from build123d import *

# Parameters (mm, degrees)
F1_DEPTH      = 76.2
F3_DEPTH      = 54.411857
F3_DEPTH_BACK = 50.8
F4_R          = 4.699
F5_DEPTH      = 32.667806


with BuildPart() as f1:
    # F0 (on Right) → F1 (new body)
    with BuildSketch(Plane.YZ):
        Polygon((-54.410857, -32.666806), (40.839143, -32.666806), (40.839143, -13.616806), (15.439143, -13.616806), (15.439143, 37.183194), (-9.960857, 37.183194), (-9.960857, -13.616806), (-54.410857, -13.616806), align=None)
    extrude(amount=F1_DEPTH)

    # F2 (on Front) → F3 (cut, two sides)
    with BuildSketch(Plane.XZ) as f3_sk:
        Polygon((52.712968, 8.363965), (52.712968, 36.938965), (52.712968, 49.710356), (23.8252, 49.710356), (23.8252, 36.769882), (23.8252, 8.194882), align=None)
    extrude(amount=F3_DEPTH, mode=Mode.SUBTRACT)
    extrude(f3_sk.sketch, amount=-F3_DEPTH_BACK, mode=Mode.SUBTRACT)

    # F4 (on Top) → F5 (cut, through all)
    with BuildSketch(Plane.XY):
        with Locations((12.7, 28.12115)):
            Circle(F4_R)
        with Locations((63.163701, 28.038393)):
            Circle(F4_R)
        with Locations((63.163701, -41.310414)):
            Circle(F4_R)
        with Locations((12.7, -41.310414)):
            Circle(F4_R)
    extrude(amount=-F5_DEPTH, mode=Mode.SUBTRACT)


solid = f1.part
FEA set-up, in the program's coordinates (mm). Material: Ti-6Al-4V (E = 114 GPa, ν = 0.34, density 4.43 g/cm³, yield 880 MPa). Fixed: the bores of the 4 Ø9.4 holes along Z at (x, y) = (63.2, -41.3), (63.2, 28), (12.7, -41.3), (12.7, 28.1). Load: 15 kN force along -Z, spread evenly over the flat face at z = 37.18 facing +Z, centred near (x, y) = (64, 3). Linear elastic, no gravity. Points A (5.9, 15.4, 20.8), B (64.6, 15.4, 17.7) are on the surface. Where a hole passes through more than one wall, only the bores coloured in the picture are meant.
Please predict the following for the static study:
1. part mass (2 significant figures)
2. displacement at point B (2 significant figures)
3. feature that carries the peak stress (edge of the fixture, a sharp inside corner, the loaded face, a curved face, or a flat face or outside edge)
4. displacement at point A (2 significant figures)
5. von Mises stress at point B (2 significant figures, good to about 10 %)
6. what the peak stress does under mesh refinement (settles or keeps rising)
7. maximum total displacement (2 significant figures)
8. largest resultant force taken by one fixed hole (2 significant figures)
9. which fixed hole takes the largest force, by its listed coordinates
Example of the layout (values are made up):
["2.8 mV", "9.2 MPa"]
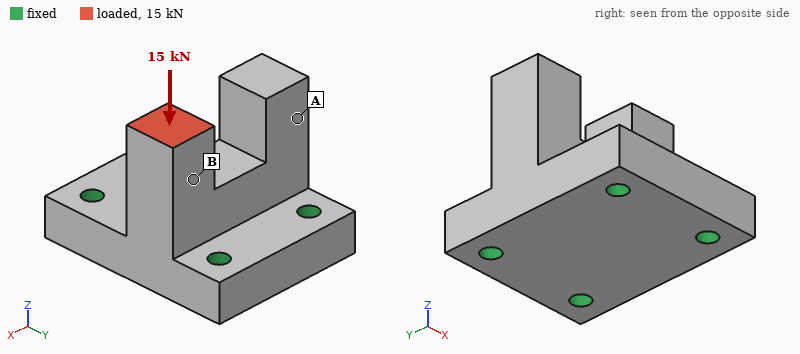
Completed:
["930 g", "22 µm", "edge of the fixture", "9.3 µm", "24 MPa", "keeps rising", "37 µm", "9.9 kN", "(63.2, 28)"]
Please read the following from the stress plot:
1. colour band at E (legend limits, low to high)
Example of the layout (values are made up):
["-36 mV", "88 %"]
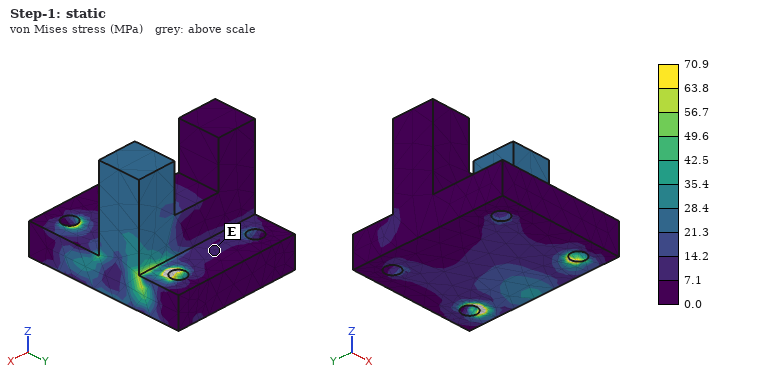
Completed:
["7.1 to 14.2 MPa"]
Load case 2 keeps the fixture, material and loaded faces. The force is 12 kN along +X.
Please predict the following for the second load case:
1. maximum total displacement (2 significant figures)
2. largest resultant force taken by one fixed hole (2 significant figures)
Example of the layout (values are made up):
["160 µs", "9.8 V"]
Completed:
["0.15 mm", "11 kN"]
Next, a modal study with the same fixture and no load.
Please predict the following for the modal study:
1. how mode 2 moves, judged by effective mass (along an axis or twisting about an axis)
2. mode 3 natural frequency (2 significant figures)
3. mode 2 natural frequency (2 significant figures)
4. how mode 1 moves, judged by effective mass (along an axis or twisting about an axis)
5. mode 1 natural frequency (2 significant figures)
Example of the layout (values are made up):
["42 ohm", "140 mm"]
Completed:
["along X", "6800 Hz", "6000 Hz", "along Y", "5600 Hz"]
